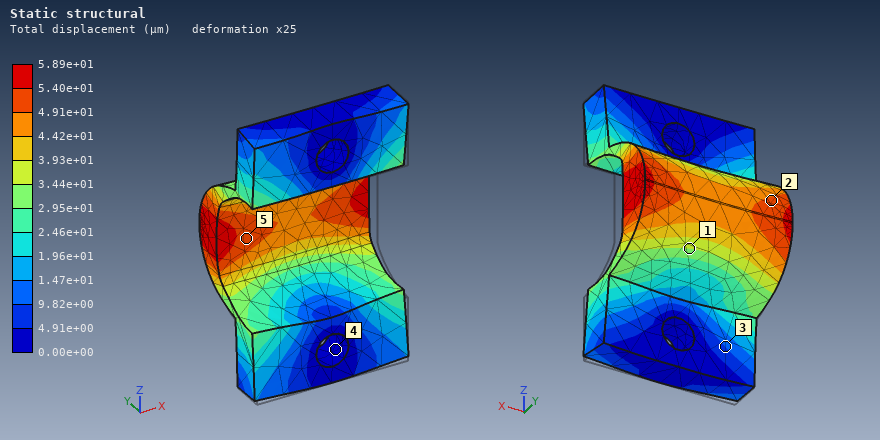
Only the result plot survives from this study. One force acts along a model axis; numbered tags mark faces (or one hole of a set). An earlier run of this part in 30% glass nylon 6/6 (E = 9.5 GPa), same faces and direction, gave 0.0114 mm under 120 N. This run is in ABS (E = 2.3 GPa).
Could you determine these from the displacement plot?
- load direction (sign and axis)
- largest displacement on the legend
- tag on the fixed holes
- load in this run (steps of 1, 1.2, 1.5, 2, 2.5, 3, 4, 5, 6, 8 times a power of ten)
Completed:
+Y
5.89e+01 µm
4
150 N
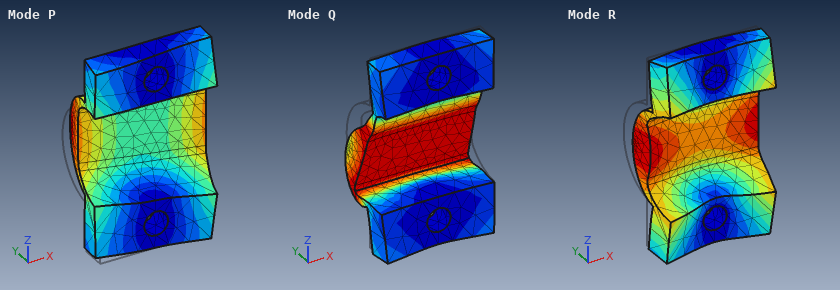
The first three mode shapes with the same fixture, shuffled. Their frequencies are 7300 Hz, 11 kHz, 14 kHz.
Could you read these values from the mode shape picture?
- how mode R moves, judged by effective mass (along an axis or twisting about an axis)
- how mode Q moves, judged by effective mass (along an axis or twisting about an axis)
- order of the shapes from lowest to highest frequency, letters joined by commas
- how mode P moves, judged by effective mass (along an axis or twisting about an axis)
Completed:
along Y
along Z
P, Q, R
along X
